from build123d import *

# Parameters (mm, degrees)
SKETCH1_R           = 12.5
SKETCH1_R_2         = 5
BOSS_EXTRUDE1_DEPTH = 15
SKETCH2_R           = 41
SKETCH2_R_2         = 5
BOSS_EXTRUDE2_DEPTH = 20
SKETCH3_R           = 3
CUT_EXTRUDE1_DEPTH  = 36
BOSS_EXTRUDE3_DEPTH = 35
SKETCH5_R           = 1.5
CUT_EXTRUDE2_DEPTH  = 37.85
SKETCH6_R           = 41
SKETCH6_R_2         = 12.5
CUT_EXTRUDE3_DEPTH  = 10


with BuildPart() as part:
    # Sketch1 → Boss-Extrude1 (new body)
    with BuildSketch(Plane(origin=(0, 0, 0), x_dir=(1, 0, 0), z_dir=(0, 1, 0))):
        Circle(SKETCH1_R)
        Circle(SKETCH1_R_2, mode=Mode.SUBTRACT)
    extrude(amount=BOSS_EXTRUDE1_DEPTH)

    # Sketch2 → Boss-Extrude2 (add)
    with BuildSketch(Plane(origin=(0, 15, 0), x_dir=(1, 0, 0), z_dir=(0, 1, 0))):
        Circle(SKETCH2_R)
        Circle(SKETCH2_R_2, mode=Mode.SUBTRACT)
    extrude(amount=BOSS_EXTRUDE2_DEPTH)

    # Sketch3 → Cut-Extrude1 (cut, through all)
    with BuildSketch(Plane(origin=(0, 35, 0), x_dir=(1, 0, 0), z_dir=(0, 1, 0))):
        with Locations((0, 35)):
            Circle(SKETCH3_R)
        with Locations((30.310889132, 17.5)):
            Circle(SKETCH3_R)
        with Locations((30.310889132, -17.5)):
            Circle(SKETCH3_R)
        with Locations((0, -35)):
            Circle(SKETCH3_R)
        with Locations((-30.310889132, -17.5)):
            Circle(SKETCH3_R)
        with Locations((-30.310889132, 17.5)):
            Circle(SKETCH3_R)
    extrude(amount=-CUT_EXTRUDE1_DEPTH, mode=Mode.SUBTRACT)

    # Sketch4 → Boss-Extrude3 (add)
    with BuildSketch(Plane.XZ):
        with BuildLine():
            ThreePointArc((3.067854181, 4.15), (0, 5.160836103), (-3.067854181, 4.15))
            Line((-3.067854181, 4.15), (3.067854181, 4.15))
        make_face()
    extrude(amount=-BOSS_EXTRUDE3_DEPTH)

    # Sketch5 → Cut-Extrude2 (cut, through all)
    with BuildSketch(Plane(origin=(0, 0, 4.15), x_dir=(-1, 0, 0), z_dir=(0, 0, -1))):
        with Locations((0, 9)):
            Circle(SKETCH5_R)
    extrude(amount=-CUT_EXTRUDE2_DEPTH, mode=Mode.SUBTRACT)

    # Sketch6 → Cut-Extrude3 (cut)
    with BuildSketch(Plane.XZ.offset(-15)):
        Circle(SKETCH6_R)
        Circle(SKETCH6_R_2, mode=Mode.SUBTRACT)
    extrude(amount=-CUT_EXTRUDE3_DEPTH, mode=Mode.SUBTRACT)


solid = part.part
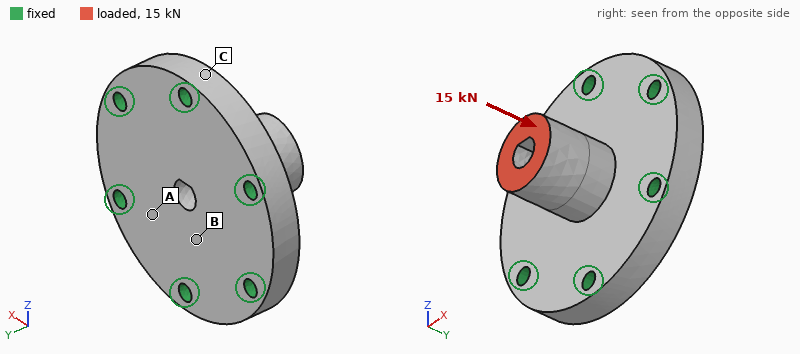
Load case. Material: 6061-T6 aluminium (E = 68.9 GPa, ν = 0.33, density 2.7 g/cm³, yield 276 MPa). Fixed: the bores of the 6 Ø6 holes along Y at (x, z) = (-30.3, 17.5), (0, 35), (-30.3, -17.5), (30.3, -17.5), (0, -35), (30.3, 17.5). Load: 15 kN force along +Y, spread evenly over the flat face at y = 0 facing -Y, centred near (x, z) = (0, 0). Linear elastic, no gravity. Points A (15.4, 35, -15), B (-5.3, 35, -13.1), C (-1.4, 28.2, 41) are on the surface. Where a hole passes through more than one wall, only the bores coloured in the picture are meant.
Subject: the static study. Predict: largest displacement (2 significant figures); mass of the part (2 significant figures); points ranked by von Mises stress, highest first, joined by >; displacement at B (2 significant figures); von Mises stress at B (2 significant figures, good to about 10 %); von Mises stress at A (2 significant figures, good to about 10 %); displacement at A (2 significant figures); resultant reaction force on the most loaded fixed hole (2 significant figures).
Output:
60 µm
160 g
B > A > C
39 µm
52 MPa
32 MPa
24 µm
2.6 kN
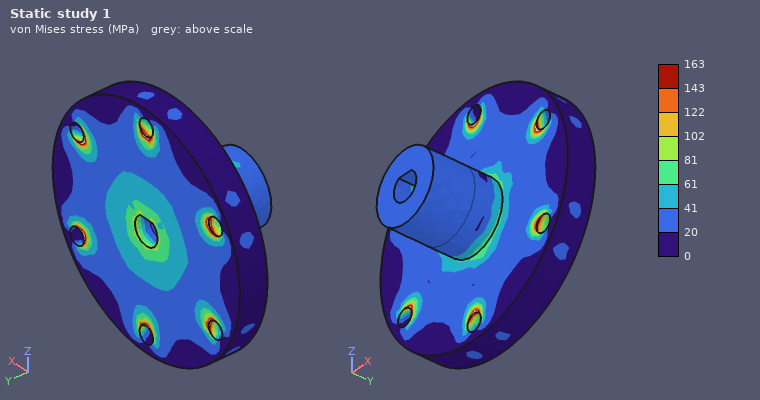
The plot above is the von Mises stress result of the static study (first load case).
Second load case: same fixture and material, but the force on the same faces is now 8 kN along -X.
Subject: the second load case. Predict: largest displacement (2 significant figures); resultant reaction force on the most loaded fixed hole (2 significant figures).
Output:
0.15 mm
3.1 kN
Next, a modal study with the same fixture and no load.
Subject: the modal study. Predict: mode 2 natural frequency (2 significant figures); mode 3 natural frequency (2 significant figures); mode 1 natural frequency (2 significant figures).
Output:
11 kHz
12 kHz
11 kHz
